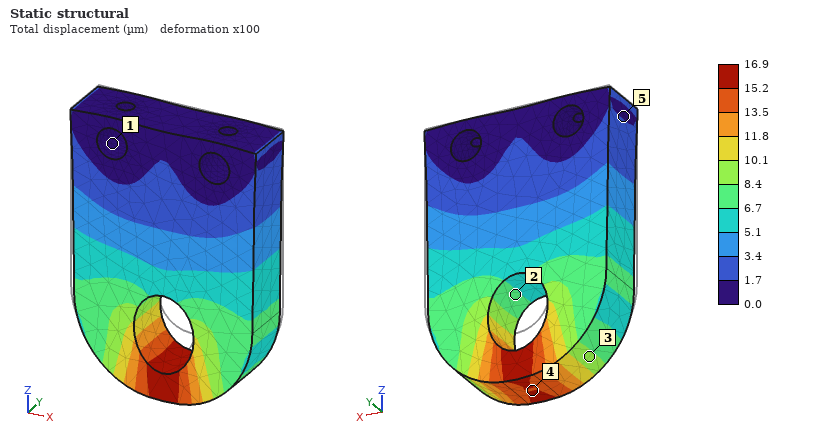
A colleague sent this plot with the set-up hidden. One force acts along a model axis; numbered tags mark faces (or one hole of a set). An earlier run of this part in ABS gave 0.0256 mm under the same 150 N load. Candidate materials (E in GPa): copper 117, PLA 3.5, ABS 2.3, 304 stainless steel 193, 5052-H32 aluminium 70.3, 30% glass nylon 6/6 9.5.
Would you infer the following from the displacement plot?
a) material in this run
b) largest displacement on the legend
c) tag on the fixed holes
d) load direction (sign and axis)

PLA
16.9 µm
1
-Z
